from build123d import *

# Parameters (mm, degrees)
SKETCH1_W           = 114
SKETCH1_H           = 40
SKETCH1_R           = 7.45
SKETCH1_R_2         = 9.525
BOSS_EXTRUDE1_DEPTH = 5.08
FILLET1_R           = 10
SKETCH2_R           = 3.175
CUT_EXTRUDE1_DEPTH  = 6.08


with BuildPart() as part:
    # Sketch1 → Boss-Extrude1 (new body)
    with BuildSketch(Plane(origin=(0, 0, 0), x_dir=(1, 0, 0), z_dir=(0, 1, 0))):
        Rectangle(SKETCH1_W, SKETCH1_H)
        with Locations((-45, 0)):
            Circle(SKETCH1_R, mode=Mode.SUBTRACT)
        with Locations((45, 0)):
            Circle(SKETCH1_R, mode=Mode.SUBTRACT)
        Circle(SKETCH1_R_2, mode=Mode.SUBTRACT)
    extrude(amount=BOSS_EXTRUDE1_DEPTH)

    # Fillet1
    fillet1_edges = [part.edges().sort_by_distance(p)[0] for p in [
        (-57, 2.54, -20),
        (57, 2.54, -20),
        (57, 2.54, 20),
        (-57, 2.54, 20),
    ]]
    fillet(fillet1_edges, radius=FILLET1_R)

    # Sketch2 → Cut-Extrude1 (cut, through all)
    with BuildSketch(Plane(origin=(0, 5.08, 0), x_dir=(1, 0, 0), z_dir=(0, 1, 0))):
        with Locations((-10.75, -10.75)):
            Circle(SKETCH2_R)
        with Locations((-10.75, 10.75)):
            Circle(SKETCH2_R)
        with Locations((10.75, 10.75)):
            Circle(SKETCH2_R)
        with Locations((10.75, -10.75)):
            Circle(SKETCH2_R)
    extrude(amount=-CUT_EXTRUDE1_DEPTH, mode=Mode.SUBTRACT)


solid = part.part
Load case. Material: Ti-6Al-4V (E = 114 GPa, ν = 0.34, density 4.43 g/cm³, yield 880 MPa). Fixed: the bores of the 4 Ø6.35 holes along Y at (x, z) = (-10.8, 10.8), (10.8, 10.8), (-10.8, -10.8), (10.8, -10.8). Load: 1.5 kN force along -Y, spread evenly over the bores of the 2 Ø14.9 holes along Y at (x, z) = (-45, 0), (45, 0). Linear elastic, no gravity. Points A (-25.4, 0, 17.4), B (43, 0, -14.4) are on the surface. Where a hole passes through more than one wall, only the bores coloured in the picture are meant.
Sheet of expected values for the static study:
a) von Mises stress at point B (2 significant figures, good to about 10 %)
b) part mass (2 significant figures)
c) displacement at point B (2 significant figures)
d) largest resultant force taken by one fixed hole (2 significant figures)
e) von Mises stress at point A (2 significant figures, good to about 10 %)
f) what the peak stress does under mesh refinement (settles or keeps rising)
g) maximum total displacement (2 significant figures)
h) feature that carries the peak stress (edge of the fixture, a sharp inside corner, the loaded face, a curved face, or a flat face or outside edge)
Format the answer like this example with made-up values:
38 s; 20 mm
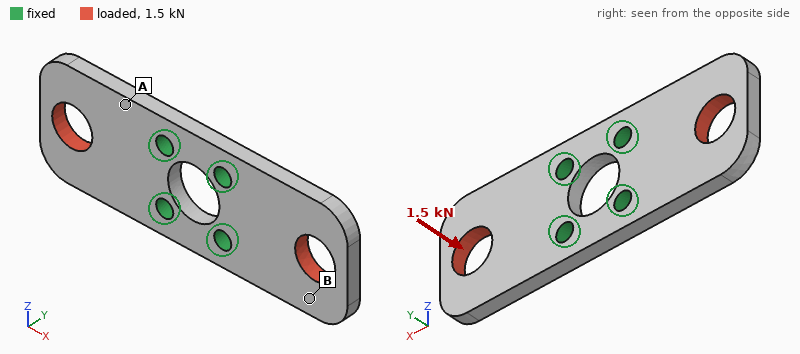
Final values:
26 MPa; 84 g; 0.16 mm; 380 N; 87 MPa; keeps rising; 0.29 mm; edge of the fixture
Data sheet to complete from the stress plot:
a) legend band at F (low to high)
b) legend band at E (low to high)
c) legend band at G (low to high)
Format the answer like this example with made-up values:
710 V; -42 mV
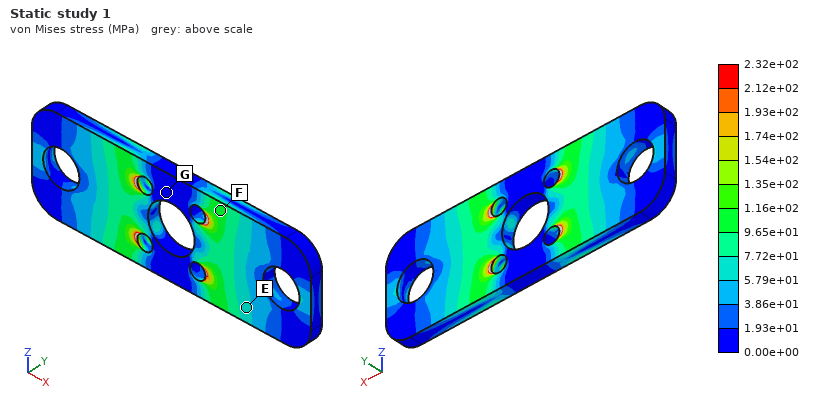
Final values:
9.65e+01 to 1.16e+02 MPa; 5.79e+01 to 7.72e+01 MPa; 0.00e+00 to 1.93e+01 MPa
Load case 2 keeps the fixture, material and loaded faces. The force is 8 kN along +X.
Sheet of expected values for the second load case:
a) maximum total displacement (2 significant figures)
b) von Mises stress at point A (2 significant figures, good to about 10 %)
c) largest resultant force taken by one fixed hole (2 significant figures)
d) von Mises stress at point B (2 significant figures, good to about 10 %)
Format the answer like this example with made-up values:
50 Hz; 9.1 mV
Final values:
15 µm; 19 MPa; 2.0 kN; 17 MPa
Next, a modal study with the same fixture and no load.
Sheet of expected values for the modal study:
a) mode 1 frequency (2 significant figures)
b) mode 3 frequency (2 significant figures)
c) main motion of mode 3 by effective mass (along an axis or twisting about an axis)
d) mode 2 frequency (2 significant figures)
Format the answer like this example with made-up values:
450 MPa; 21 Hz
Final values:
2400 Hz; 5300 Hz; twisting about X; 2400 Hz
